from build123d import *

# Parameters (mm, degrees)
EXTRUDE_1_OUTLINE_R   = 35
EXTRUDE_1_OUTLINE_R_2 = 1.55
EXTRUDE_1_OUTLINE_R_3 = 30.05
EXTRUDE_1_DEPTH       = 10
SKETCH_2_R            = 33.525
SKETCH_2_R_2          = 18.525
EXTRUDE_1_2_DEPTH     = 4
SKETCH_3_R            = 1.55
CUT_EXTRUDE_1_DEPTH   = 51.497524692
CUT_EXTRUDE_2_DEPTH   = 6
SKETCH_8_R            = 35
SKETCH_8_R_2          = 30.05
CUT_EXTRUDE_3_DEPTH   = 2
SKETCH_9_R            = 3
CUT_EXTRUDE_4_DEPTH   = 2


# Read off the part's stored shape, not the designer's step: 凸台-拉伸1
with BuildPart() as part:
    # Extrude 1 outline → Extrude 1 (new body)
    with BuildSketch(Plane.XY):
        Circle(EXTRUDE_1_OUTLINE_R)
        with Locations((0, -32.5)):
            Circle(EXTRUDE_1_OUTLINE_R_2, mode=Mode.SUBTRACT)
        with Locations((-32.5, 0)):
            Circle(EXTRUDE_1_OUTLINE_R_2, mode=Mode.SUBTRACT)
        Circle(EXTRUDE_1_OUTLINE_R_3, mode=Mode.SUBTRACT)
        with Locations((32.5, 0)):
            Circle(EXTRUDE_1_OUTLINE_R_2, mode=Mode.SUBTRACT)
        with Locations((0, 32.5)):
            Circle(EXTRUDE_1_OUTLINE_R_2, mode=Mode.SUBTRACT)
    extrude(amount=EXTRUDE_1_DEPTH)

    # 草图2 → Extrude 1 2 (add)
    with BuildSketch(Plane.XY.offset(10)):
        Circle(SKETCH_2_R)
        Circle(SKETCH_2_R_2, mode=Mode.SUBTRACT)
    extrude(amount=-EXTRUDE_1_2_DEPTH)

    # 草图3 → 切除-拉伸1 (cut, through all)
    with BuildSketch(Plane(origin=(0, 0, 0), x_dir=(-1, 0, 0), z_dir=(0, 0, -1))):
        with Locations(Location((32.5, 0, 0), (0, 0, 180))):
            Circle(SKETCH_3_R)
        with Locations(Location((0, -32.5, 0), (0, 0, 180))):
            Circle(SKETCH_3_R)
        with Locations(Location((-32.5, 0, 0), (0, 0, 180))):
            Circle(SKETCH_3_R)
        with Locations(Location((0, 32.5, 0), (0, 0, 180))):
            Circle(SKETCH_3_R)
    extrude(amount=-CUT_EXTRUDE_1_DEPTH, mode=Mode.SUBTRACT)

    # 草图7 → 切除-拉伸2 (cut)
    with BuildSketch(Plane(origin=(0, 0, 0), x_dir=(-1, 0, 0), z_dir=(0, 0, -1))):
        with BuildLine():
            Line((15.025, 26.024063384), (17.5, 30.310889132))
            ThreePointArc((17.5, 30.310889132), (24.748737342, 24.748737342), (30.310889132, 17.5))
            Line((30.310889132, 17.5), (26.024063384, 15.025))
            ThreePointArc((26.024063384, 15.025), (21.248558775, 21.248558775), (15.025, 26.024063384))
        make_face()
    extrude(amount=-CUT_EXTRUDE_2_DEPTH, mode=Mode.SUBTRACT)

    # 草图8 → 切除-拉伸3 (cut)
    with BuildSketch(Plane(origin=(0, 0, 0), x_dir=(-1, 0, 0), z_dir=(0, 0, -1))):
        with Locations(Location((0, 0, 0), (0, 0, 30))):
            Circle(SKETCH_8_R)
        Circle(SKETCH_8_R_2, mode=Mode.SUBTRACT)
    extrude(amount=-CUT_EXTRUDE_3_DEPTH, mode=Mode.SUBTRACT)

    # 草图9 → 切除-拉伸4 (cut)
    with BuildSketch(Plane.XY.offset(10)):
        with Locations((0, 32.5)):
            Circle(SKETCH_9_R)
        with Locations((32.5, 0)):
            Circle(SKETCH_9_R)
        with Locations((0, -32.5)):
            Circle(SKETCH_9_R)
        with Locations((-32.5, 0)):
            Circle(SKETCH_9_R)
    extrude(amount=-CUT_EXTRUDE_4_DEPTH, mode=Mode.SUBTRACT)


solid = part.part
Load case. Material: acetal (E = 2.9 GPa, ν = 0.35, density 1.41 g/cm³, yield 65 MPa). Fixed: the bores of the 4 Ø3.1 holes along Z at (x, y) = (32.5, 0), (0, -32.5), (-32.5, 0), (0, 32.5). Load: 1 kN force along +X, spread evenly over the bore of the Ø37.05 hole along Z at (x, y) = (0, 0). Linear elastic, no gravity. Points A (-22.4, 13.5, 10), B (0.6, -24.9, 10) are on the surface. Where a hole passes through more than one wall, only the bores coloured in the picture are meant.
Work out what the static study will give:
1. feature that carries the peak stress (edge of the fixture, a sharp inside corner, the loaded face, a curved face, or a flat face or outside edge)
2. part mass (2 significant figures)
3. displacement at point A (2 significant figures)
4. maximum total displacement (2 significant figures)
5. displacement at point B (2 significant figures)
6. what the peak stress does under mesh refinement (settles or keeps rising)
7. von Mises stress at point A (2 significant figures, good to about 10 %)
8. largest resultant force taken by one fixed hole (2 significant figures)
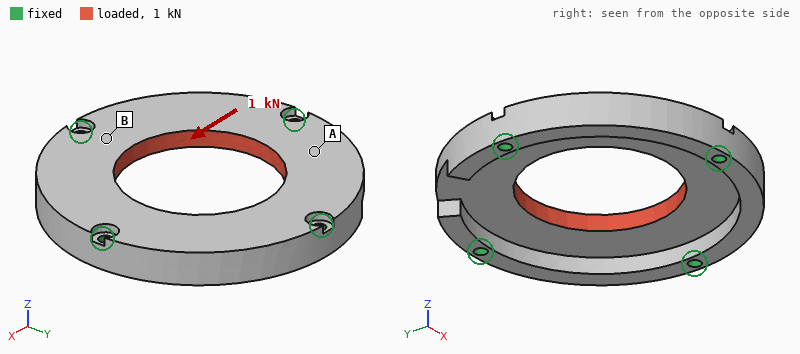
edge of the fixture
20 g
44 µm
61 µm
26 µm
keeps rising
2.9 MPa
270 N
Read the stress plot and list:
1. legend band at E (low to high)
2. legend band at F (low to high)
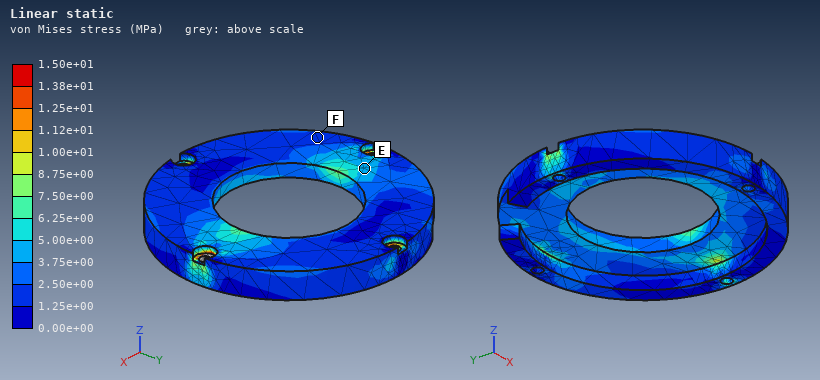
3.75e+00 to 5.00e+00 MPa
1.25e+00 to 2.50e+00 MPa
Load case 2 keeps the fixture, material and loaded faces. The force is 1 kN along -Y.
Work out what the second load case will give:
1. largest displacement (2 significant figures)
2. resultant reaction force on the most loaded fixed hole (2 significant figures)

61 µm
270 N
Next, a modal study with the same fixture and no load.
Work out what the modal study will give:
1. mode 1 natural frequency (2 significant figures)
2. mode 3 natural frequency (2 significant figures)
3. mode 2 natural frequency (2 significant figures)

3000 Hz
3200 Hz
3100 Hz
